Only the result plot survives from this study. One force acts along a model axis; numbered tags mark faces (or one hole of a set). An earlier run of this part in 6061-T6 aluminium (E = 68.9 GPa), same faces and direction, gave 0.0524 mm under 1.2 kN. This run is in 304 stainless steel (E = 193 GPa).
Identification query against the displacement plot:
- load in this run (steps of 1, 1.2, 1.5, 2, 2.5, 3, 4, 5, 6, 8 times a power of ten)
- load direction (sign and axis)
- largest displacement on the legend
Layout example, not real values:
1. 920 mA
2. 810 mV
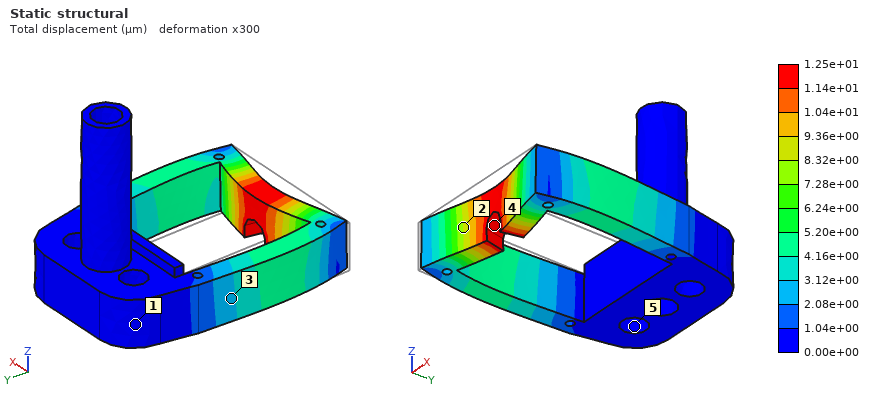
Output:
1. 800 N
2. +Y
3. 1.25e+01 µm
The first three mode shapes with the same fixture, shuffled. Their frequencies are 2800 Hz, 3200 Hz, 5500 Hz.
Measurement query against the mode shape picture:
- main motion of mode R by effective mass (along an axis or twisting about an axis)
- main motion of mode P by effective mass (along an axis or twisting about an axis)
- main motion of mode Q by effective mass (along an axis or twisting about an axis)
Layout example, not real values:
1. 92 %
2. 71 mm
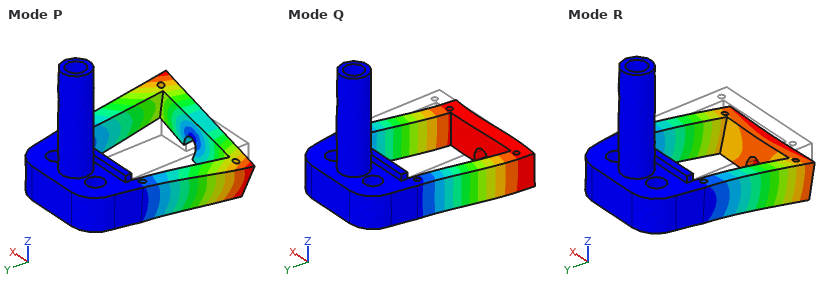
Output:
1. along Z
2. twisting about Y
3. along X
